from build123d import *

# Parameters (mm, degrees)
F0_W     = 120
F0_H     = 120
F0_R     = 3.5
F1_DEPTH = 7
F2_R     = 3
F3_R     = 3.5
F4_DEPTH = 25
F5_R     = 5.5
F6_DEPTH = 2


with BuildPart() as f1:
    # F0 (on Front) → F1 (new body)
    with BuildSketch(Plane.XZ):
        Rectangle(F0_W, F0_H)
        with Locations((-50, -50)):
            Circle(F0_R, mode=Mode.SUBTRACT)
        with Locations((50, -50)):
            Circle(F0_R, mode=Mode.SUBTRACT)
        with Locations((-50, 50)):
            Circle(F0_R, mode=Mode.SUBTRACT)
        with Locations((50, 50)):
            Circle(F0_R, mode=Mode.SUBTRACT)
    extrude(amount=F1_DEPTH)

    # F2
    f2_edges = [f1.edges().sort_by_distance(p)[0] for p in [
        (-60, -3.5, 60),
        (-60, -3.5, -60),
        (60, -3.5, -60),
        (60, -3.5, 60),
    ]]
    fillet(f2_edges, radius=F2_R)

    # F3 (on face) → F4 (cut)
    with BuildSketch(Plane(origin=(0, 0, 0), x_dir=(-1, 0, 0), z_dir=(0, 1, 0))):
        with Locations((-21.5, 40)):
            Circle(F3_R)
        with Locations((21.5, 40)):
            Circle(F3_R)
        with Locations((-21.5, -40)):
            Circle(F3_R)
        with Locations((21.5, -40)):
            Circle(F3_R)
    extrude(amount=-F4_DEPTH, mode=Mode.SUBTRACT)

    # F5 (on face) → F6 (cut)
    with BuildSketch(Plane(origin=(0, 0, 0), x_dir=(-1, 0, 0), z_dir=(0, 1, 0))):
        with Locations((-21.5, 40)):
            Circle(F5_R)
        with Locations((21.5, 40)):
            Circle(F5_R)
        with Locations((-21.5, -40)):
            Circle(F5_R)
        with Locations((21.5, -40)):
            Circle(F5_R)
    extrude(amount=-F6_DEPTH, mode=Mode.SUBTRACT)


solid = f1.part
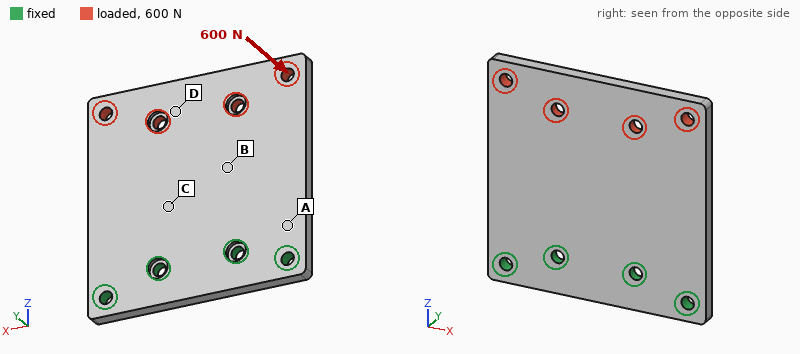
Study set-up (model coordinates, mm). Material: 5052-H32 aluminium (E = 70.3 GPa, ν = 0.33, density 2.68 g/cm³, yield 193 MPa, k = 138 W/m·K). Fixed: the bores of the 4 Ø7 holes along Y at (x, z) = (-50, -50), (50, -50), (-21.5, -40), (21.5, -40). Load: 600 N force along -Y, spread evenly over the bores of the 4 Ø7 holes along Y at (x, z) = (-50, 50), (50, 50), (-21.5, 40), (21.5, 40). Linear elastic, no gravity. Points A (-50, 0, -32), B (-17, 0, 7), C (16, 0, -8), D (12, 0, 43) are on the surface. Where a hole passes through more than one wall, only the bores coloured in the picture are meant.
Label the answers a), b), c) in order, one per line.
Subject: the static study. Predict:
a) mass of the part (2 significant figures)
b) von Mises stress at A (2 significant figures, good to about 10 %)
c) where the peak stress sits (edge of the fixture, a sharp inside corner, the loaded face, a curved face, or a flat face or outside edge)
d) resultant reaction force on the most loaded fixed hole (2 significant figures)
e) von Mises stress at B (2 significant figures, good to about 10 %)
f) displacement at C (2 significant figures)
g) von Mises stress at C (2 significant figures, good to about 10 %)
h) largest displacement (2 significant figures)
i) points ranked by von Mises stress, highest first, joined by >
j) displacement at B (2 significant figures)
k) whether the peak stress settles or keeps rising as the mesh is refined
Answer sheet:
a) 260 g
b) 41 MPa
c) edge of the fixture
d) 620 N
e) 20 MPa
f) 0.13 mm
g) 28 MPa
h) 0.74 mm
i) A > C > B > D
j) 0.24 mm
k) keeps rising
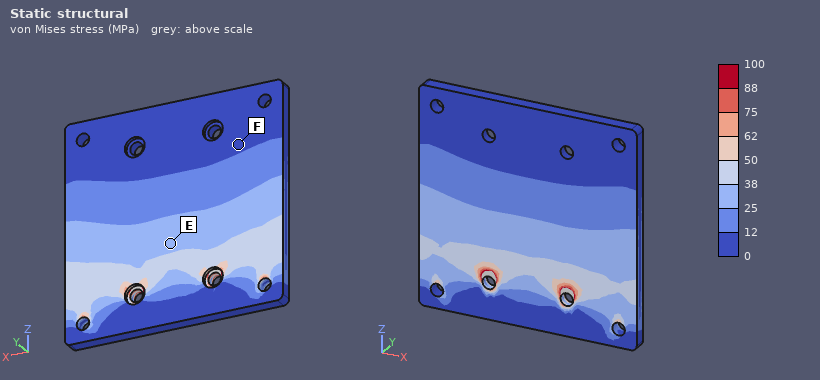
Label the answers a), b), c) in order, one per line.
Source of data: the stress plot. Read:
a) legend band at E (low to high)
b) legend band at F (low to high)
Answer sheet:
a) 25 to 38 MPa
b) 0 to 12 MPa
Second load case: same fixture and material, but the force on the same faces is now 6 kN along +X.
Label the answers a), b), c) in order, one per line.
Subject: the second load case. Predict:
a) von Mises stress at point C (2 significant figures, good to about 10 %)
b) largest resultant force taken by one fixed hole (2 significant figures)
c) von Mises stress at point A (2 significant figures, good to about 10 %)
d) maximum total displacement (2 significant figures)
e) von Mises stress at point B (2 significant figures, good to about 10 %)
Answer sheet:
a) 16 MPa
b) 4.4 kN
c) 28 MPa
d) 74 µm
e) 16 MPa
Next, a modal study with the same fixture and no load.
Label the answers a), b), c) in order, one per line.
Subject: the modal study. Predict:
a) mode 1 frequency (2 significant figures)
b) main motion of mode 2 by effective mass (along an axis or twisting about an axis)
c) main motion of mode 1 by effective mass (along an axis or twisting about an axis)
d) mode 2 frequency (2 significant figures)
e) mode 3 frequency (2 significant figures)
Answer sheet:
a) 550 Hz
b) twisting about Z
c) along Y
d) 1200 Hz
e) 3000 Hz
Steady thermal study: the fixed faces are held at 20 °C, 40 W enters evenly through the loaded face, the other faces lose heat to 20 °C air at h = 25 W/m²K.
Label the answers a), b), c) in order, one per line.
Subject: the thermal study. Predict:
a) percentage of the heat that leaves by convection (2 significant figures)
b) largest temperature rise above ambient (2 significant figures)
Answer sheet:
a) 25 %
b) 31 K
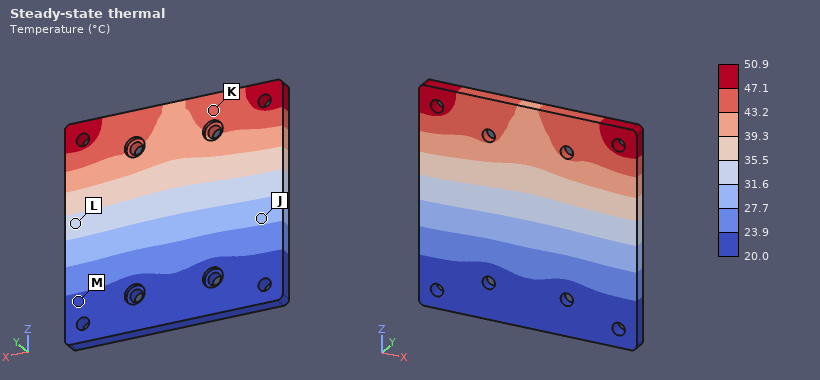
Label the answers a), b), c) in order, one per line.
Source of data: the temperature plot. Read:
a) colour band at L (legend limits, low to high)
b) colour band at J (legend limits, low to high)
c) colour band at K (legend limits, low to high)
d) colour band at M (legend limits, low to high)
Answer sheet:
a) 31.6 to 35.5 °C
b) 27.7 to 31.6 °C
c) 43.2 to 47.1 °C
d) 20.0 to 23.9 °C
